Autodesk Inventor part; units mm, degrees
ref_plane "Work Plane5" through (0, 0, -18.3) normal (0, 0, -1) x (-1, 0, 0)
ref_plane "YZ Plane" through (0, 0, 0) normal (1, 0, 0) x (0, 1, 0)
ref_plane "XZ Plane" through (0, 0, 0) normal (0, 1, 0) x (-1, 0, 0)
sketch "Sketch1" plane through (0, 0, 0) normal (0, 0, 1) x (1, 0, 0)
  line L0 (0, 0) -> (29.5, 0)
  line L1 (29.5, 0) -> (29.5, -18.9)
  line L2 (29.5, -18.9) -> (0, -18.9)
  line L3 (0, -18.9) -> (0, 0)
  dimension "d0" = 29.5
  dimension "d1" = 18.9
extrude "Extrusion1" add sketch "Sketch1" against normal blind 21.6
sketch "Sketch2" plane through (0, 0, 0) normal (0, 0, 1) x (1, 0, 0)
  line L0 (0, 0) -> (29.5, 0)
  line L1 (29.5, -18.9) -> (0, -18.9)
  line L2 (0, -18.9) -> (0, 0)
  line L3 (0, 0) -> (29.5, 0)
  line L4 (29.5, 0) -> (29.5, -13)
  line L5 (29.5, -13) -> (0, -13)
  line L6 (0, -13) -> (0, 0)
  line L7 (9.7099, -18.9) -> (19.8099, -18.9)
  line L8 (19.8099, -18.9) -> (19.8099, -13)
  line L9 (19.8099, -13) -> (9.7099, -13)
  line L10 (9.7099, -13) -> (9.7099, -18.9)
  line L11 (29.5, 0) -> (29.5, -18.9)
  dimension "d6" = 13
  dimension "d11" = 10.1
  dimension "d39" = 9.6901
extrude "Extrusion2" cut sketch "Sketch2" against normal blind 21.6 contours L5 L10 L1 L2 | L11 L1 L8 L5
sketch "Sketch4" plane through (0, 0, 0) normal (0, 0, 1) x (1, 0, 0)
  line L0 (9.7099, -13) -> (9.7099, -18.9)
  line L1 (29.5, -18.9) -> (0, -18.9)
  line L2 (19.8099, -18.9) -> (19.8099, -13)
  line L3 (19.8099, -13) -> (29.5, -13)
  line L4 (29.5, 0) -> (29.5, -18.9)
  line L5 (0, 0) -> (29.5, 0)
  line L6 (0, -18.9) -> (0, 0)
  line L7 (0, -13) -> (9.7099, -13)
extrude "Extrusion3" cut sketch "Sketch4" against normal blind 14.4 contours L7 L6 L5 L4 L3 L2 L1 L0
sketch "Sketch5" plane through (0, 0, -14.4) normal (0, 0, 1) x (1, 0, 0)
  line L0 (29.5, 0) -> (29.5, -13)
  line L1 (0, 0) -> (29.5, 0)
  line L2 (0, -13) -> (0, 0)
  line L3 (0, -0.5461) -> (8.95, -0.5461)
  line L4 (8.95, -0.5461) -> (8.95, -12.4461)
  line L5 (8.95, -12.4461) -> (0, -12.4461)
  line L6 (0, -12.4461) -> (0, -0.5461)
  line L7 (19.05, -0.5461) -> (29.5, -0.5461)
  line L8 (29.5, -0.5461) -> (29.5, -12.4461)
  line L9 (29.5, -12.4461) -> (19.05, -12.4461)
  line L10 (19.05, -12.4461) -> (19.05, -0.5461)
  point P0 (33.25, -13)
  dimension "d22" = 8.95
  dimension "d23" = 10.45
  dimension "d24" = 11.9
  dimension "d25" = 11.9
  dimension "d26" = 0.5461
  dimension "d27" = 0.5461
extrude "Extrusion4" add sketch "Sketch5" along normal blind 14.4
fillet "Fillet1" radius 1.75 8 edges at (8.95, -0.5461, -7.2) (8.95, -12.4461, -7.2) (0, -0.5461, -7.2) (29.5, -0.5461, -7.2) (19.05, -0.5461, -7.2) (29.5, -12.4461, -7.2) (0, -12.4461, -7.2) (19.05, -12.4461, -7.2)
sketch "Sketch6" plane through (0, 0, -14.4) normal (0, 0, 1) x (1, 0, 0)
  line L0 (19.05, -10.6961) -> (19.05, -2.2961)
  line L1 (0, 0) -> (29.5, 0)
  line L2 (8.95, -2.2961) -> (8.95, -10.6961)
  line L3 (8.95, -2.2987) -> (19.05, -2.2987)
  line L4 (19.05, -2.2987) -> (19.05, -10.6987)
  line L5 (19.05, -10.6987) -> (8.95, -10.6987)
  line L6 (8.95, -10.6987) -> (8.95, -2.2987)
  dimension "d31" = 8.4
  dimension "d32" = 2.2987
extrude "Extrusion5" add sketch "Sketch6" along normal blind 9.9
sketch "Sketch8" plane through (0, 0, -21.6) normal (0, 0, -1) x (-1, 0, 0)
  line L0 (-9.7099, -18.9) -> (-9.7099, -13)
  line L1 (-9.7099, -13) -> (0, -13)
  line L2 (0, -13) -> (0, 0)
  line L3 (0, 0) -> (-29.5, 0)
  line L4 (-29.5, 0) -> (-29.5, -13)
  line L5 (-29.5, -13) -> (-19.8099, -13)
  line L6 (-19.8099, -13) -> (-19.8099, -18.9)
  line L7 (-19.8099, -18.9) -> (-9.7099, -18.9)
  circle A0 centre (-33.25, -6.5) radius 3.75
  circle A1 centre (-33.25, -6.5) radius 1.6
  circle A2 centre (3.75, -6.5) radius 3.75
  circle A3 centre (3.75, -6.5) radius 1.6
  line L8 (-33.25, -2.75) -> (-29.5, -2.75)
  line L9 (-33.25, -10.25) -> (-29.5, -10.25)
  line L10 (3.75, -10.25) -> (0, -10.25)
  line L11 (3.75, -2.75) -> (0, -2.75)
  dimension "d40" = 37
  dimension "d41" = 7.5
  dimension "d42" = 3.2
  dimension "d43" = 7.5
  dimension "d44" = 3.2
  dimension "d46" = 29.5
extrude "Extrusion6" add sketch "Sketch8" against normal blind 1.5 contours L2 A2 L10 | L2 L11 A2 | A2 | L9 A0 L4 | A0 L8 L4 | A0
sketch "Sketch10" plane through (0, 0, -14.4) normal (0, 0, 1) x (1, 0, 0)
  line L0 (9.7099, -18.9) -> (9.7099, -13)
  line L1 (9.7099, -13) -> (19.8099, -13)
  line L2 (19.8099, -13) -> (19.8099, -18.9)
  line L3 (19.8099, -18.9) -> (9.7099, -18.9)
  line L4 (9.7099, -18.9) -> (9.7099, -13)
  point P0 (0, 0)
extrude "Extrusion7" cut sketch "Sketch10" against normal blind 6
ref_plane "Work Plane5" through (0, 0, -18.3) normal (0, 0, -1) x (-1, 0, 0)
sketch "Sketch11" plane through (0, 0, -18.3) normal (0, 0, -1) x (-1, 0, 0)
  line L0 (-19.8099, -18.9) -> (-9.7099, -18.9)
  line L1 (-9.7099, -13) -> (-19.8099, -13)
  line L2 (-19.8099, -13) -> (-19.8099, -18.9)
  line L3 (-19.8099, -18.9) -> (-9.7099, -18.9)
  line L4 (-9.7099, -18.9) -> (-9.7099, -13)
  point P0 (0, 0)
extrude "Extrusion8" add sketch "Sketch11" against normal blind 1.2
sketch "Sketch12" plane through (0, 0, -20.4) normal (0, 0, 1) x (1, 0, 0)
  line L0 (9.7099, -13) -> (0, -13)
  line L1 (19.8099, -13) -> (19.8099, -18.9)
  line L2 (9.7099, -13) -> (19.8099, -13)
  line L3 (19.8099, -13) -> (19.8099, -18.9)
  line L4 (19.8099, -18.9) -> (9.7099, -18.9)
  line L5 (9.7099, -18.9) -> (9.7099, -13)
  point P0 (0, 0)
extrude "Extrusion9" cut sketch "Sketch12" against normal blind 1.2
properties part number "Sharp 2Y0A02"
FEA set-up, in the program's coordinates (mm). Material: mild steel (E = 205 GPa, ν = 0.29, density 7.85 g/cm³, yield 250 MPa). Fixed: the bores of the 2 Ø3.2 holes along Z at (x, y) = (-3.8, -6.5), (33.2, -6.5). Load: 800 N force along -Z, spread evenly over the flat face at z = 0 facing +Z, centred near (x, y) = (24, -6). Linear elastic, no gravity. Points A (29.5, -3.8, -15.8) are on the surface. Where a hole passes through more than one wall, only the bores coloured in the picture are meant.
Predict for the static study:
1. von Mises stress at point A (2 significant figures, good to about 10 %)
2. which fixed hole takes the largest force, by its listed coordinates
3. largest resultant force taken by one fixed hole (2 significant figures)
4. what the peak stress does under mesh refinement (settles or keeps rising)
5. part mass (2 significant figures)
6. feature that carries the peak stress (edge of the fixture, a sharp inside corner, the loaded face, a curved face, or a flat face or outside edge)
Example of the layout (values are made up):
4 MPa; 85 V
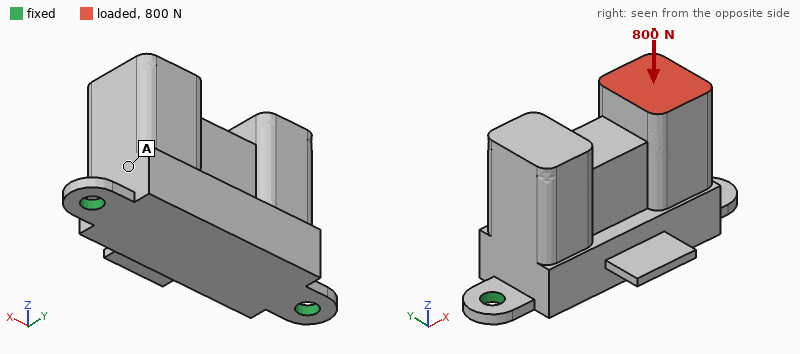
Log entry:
23 MPa; (33.2, -6.5); 670 N; keeps rising; 55 g; edge of the fixture
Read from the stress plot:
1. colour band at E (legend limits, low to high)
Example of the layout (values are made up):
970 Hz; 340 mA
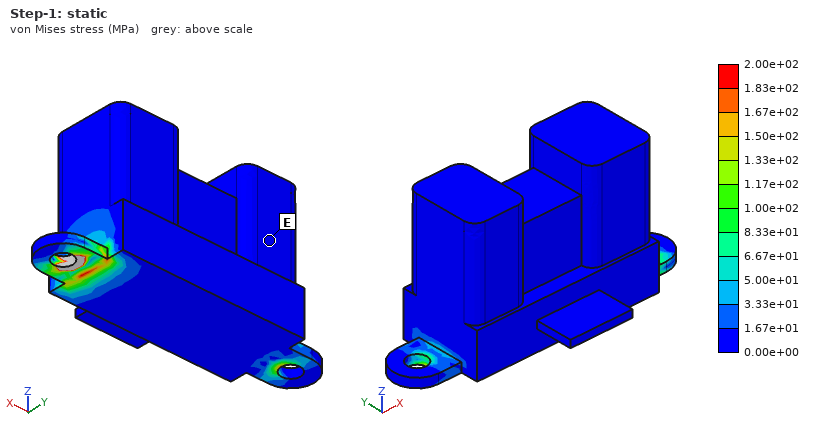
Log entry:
0.00e+00 to 1.67e+01 MPa
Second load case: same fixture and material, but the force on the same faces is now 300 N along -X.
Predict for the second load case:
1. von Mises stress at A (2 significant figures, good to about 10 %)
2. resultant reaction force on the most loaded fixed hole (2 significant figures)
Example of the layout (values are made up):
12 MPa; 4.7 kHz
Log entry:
7.6 MPa; 260 N
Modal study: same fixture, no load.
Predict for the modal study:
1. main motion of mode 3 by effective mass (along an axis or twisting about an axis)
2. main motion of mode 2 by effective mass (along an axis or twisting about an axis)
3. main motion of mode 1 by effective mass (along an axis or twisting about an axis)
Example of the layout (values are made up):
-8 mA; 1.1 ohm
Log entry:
along X; along Z; along Y
